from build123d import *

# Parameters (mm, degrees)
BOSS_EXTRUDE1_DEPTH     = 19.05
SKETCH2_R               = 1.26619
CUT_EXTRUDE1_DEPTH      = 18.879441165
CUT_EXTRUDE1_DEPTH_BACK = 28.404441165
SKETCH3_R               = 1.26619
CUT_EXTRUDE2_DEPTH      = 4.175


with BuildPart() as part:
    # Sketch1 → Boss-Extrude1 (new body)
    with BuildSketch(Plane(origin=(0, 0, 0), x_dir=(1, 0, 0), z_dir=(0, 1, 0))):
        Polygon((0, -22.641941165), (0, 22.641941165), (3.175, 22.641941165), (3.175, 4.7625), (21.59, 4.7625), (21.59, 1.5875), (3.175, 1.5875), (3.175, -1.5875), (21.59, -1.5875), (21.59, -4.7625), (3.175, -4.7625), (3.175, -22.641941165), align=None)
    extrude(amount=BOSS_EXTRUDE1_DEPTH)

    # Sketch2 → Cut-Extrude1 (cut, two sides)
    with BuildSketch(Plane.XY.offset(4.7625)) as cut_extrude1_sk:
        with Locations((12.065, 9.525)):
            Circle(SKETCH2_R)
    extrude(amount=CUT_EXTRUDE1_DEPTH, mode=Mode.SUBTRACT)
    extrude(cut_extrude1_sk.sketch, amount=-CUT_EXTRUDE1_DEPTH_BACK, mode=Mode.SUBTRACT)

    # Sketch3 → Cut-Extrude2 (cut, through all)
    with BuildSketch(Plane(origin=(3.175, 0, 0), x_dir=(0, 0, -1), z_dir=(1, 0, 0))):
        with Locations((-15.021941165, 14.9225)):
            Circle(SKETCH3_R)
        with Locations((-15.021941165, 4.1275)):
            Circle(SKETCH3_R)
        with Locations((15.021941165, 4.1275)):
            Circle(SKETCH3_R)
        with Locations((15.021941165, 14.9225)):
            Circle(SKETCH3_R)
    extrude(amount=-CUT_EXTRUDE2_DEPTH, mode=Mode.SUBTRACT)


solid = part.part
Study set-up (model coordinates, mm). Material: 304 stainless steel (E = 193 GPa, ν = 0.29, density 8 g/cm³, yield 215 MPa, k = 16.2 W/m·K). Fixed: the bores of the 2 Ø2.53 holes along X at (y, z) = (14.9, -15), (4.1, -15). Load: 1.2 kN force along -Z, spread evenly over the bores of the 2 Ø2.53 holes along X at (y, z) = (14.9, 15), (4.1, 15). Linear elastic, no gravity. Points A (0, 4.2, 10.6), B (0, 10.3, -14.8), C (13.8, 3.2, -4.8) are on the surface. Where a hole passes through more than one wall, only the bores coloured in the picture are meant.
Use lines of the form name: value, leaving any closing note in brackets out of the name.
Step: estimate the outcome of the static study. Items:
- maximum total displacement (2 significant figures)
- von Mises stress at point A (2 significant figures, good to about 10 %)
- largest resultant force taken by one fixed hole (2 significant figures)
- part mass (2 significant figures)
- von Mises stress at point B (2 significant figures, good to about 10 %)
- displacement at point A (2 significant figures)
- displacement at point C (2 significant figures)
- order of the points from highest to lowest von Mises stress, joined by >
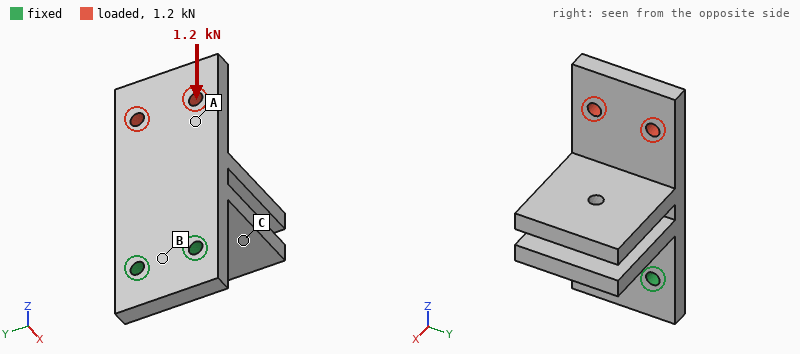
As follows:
maximum total displacement: 4.3 µm
von Mises stress at point A: 23 MPa
largest resultant force taken by one fixed hole: 600 N
part mass: 39 g
von Mises stress at point B: 8.3 MPa
displacement at point A: 3.2 µm
displacement at point C: 0.92 µm
order of the points from highest to lowest von Mises stress, joined by >: A > B > C
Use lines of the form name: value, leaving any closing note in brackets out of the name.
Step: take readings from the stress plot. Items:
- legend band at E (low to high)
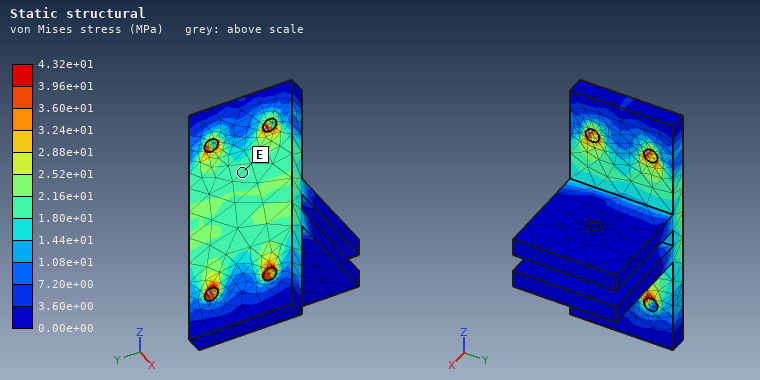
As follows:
legend band at E: 1.80e+01 to 2.16e+01 MPa
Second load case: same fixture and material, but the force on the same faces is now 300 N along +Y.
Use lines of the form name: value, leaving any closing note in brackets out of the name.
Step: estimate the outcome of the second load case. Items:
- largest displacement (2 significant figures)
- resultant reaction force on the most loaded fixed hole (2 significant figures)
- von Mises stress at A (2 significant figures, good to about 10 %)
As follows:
largest displacement: 14 µm
resultant reaction force on the most loaded fixed hole: 750 N
von Mises stress at A: 11 MPa
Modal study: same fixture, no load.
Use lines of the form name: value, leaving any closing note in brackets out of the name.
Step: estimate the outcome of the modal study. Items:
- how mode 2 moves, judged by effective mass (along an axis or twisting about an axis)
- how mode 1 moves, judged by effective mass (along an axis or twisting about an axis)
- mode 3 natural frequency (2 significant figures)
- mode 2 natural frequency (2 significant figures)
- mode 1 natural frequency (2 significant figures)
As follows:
how mode 2 moves, judged by effective mass: along Y
how mode 1 moves, judged by effective mass: along X
mode 3 natural frequency: 5300 Hz
mode 2 natural frequency: 3800 Hz
mode 1 natural frequency: 1400 Hz
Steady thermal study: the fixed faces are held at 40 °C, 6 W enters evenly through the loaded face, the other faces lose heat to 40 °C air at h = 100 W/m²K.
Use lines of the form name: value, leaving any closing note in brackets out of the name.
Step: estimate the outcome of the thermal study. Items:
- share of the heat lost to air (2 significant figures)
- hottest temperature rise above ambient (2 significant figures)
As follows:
share of the heat lost to air: 90 %
hottest temperature rise above ambient: 59 K
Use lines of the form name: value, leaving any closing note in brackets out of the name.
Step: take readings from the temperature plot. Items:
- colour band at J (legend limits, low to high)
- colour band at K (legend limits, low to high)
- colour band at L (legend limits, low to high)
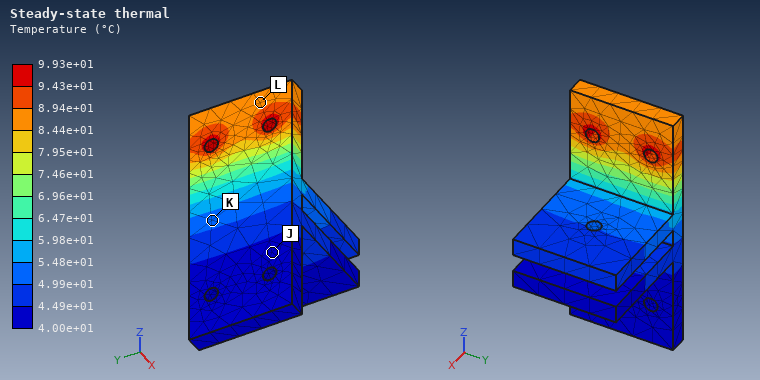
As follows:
colour band at J: 4.00e+01 to 4.49e+01 °C
colour band at K: 4.99e+01 to 5.48e+01 °C
colour band at L: 8.44e+01 to 8.94e+01 °C
